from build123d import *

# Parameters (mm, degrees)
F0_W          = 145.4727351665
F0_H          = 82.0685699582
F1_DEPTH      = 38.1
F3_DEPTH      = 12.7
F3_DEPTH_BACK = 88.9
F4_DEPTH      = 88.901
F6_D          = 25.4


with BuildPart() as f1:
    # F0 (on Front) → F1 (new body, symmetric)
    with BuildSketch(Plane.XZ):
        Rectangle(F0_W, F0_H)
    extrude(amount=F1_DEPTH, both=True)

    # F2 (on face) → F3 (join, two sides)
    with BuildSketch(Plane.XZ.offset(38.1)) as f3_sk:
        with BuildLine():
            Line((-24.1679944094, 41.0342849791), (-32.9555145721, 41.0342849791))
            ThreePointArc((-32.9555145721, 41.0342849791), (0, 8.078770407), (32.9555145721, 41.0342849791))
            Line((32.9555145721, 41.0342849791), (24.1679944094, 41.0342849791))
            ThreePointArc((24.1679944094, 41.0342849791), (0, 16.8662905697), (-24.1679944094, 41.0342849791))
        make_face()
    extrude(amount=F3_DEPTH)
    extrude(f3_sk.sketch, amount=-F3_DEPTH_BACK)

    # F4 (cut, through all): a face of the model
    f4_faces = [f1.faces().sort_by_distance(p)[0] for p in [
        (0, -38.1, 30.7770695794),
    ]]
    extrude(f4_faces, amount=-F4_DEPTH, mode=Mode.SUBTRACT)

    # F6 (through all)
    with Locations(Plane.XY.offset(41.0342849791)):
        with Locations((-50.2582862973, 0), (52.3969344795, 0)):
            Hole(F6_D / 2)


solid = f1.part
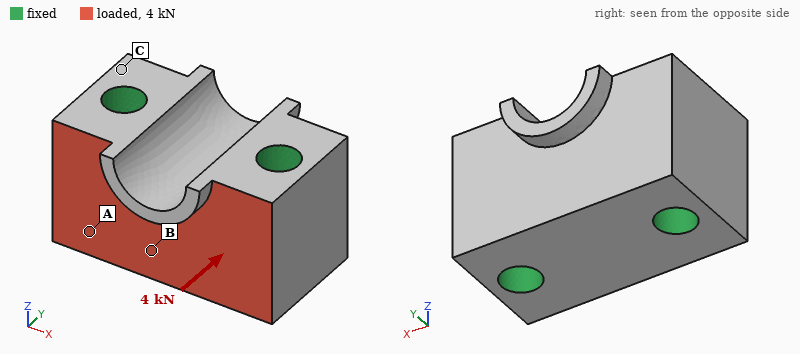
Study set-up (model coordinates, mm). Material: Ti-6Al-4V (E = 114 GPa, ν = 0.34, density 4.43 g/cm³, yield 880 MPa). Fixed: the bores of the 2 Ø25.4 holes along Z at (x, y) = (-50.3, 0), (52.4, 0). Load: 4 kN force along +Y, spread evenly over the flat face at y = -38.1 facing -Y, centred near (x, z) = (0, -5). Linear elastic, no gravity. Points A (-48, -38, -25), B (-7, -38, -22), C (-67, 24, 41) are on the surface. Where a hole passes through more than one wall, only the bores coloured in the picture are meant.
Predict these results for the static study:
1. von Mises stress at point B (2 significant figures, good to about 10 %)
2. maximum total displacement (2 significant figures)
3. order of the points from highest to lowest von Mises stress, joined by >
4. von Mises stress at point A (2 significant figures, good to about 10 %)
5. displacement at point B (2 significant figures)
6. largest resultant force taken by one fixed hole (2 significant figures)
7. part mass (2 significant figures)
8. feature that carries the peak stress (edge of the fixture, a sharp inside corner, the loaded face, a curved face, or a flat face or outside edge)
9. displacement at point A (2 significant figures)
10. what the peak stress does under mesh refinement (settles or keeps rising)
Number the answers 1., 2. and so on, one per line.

1. 0.33 MPa
2. 0.29 µm
3. A > B > C
4. 0.52 MPa
5. 0.24 µm
6. 2.0 kN
7. 3.4 kg
8. edge of the fixture
9. 0.12 µm
10. keeps rising
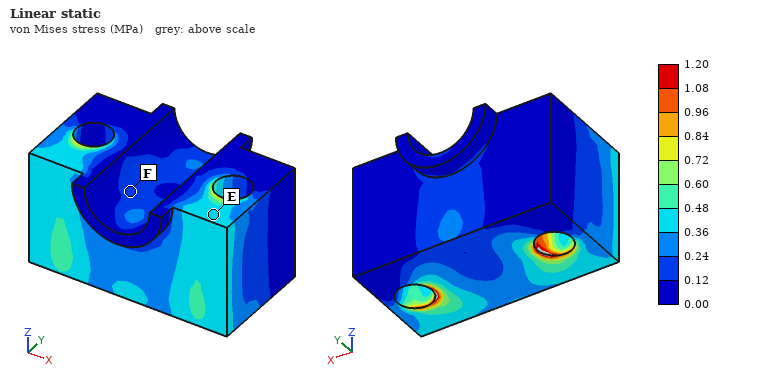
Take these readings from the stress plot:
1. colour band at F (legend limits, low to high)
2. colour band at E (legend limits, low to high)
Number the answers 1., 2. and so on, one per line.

1. 0.12 to 0.24 MPa
2. 0.36 to 0.48 MPa
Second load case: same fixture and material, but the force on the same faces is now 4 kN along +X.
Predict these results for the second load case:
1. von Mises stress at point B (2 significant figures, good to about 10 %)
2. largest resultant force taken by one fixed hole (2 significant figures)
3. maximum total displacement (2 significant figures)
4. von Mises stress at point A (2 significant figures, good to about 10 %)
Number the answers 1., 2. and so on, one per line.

1. 0.68 MPa
2. 2.2 kN
3. 0.59 µm
4. 0.80 MPa
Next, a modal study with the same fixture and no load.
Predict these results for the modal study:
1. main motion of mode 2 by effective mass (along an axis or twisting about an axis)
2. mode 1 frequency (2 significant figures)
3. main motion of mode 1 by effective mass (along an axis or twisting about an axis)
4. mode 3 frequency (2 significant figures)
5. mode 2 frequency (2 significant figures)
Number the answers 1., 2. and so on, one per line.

1. along Z
2. 14 kHz
3. along Y
4. 16 kHz
5. 14 kHz
